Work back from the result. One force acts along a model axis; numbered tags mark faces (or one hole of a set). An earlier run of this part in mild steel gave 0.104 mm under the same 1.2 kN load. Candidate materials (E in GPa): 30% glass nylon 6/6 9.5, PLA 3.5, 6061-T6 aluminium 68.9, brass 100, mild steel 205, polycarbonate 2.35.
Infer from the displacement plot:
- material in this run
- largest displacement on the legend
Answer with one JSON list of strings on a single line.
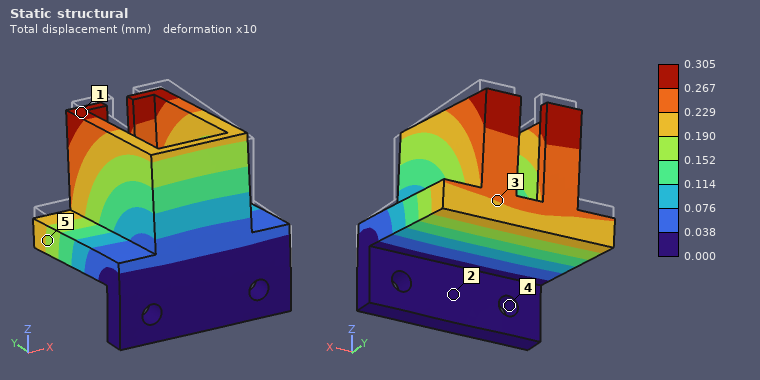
["6061-T6 aluminium", "0.305 mm"]
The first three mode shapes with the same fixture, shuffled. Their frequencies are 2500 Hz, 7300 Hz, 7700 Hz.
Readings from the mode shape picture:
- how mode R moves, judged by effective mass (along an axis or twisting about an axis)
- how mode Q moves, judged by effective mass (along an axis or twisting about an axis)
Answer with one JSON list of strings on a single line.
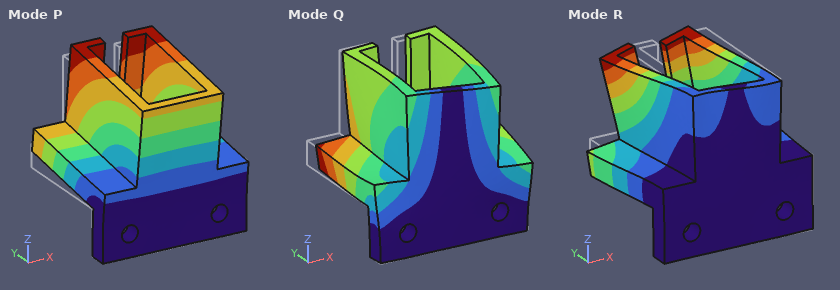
["along X", "along X"]
